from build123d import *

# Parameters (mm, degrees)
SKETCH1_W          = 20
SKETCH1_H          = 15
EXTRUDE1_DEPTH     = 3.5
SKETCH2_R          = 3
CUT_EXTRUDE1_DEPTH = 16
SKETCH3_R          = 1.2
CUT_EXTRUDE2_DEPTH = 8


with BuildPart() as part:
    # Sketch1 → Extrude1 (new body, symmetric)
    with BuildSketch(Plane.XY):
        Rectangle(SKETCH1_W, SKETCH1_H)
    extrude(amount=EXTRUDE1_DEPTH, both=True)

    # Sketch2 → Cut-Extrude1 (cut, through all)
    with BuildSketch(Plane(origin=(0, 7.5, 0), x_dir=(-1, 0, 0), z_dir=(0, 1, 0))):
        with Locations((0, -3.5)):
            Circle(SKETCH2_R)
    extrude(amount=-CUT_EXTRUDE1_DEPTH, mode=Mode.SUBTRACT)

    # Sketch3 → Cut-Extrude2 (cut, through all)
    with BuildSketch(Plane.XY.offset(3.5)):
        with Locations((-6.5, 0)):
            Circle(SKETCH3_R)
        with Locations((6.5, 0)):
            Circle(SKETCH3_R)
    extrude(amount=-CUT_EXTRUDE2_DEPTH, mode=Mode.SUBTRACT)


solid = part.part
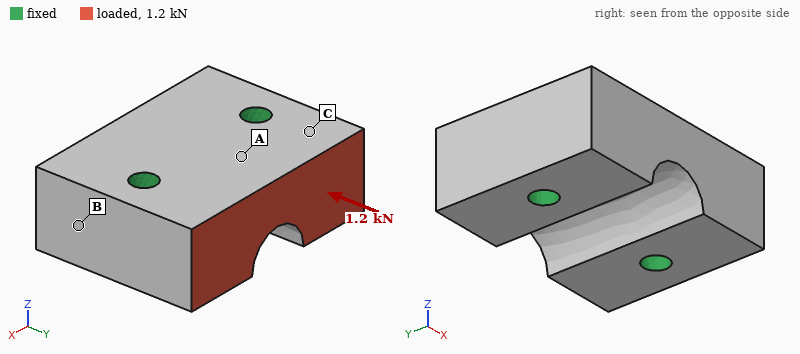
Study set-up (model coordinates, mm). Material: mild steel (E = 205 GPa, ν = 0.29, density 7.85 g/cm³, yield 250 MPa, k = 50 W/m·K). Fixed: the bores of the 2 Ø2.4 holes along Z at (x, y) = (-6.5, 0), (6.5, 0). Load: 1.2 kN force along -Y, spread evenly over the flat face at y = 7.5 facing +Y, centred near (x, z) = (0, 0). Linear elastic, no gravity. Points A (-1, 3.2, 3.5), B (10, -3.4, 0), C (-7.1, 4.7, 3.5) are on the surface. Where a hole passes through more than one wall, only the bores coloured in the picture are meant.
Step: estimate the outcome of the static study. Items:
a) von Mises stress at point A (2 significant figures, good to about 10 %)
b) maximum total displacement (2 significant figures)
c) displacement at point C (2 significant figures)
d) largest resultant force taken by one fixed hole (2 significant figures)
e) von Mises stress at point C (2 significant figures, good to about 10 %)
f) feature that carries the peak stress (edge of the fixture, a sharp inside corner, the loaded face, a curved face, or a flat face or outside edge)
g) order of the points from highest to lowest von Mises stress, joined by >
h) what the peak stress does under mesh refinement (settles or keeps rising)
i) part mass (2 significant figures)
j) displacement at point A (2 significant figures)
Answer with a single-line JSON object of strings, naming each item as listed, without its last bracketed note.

{"von Mises stress at point A": "6.2 MPa", "maximum total displacement": "0.53 µm", "displacement at point C": "0.27 µm", "largest resultant force taken by one fixed hole": "600 N", "von Mises stress at point C": "11 MPa", "feature that carries the peak stress": "edge of the fixture", "order of the points from highest to lowest von Mises stress, joined by >": "C > A > B", "what the peak stress does under mesh refinement": "keeps rising", "part mass": "14 g", "displacement at point A": "0.34 µm"}
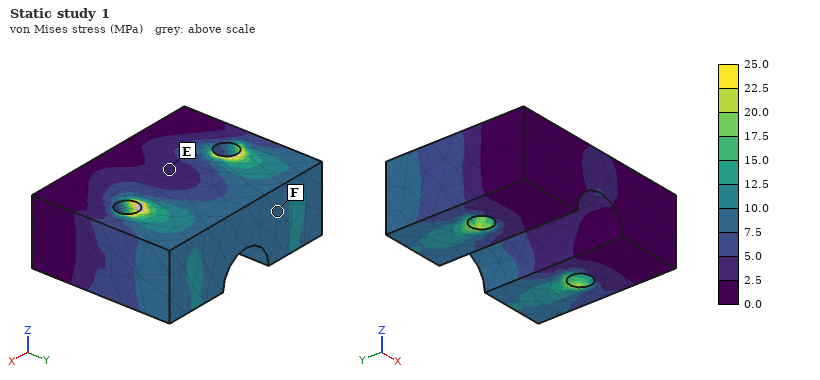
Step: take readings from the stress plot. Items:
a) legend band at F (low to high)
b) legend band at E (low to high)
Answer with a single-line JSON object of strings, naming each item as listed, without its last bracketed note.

{"legend band at F": "7.5 to 10.0 MPa", "legend band at E": "2.5 to 5.0 MPa"}
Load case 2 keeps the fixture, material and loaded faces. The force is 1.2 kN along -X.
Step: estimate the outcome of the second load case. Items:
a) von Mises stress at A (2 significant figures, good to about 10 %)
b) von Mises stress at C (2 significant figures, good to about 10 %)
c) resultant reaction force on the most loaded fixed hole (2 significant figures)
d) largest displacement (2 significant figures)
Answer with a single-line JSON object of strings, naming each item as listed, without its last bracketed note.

{"von Mises stress at A": "23 MPa", "von Mises stress at C": "14 MPa", "resultant reaction force on the most loaded fixed hole": "810 N", "largest displacement": "2.2 µm"}
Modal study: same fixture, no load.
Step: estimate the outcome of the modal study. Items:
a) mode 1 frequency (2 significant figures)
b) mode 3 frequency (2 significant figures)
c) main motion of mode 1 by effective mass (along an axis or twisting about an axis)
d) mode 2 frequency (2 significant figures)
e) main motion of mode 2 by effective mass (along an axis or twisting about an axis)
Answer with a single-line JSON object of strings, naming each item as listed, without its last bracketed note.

{"mode 1 frequency": "59 kHz", "mode 3 frequency": "72 kHz", "main motion of mode 1 by effective mass": "twisting about X", "mode 2 frequency": "69 kHz", "main motion of mode 2 by effective mass": "along Z"}
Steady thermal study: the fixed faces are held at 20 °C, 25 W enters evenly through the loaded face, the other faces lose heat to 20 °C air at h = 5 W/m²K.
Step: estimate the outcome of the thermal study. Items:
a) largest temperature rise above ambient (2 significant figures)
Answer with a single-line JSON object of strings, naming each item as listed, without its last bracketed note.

{"largest temperature rise above ambient": "32 K"}
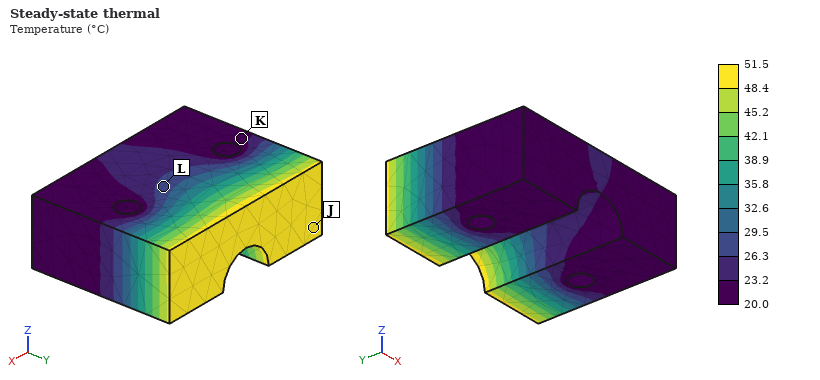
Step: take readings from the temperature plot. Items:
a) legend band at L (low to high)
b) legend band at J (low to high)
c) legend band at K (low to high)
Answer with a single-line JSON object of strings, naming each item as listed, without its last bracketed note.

{"legend band at L": "26.3 to 29.5 °C", "legend band at J": "48.4 to 51.5 °C", "legend band at K": "20.0 to 23.2 °C"}
